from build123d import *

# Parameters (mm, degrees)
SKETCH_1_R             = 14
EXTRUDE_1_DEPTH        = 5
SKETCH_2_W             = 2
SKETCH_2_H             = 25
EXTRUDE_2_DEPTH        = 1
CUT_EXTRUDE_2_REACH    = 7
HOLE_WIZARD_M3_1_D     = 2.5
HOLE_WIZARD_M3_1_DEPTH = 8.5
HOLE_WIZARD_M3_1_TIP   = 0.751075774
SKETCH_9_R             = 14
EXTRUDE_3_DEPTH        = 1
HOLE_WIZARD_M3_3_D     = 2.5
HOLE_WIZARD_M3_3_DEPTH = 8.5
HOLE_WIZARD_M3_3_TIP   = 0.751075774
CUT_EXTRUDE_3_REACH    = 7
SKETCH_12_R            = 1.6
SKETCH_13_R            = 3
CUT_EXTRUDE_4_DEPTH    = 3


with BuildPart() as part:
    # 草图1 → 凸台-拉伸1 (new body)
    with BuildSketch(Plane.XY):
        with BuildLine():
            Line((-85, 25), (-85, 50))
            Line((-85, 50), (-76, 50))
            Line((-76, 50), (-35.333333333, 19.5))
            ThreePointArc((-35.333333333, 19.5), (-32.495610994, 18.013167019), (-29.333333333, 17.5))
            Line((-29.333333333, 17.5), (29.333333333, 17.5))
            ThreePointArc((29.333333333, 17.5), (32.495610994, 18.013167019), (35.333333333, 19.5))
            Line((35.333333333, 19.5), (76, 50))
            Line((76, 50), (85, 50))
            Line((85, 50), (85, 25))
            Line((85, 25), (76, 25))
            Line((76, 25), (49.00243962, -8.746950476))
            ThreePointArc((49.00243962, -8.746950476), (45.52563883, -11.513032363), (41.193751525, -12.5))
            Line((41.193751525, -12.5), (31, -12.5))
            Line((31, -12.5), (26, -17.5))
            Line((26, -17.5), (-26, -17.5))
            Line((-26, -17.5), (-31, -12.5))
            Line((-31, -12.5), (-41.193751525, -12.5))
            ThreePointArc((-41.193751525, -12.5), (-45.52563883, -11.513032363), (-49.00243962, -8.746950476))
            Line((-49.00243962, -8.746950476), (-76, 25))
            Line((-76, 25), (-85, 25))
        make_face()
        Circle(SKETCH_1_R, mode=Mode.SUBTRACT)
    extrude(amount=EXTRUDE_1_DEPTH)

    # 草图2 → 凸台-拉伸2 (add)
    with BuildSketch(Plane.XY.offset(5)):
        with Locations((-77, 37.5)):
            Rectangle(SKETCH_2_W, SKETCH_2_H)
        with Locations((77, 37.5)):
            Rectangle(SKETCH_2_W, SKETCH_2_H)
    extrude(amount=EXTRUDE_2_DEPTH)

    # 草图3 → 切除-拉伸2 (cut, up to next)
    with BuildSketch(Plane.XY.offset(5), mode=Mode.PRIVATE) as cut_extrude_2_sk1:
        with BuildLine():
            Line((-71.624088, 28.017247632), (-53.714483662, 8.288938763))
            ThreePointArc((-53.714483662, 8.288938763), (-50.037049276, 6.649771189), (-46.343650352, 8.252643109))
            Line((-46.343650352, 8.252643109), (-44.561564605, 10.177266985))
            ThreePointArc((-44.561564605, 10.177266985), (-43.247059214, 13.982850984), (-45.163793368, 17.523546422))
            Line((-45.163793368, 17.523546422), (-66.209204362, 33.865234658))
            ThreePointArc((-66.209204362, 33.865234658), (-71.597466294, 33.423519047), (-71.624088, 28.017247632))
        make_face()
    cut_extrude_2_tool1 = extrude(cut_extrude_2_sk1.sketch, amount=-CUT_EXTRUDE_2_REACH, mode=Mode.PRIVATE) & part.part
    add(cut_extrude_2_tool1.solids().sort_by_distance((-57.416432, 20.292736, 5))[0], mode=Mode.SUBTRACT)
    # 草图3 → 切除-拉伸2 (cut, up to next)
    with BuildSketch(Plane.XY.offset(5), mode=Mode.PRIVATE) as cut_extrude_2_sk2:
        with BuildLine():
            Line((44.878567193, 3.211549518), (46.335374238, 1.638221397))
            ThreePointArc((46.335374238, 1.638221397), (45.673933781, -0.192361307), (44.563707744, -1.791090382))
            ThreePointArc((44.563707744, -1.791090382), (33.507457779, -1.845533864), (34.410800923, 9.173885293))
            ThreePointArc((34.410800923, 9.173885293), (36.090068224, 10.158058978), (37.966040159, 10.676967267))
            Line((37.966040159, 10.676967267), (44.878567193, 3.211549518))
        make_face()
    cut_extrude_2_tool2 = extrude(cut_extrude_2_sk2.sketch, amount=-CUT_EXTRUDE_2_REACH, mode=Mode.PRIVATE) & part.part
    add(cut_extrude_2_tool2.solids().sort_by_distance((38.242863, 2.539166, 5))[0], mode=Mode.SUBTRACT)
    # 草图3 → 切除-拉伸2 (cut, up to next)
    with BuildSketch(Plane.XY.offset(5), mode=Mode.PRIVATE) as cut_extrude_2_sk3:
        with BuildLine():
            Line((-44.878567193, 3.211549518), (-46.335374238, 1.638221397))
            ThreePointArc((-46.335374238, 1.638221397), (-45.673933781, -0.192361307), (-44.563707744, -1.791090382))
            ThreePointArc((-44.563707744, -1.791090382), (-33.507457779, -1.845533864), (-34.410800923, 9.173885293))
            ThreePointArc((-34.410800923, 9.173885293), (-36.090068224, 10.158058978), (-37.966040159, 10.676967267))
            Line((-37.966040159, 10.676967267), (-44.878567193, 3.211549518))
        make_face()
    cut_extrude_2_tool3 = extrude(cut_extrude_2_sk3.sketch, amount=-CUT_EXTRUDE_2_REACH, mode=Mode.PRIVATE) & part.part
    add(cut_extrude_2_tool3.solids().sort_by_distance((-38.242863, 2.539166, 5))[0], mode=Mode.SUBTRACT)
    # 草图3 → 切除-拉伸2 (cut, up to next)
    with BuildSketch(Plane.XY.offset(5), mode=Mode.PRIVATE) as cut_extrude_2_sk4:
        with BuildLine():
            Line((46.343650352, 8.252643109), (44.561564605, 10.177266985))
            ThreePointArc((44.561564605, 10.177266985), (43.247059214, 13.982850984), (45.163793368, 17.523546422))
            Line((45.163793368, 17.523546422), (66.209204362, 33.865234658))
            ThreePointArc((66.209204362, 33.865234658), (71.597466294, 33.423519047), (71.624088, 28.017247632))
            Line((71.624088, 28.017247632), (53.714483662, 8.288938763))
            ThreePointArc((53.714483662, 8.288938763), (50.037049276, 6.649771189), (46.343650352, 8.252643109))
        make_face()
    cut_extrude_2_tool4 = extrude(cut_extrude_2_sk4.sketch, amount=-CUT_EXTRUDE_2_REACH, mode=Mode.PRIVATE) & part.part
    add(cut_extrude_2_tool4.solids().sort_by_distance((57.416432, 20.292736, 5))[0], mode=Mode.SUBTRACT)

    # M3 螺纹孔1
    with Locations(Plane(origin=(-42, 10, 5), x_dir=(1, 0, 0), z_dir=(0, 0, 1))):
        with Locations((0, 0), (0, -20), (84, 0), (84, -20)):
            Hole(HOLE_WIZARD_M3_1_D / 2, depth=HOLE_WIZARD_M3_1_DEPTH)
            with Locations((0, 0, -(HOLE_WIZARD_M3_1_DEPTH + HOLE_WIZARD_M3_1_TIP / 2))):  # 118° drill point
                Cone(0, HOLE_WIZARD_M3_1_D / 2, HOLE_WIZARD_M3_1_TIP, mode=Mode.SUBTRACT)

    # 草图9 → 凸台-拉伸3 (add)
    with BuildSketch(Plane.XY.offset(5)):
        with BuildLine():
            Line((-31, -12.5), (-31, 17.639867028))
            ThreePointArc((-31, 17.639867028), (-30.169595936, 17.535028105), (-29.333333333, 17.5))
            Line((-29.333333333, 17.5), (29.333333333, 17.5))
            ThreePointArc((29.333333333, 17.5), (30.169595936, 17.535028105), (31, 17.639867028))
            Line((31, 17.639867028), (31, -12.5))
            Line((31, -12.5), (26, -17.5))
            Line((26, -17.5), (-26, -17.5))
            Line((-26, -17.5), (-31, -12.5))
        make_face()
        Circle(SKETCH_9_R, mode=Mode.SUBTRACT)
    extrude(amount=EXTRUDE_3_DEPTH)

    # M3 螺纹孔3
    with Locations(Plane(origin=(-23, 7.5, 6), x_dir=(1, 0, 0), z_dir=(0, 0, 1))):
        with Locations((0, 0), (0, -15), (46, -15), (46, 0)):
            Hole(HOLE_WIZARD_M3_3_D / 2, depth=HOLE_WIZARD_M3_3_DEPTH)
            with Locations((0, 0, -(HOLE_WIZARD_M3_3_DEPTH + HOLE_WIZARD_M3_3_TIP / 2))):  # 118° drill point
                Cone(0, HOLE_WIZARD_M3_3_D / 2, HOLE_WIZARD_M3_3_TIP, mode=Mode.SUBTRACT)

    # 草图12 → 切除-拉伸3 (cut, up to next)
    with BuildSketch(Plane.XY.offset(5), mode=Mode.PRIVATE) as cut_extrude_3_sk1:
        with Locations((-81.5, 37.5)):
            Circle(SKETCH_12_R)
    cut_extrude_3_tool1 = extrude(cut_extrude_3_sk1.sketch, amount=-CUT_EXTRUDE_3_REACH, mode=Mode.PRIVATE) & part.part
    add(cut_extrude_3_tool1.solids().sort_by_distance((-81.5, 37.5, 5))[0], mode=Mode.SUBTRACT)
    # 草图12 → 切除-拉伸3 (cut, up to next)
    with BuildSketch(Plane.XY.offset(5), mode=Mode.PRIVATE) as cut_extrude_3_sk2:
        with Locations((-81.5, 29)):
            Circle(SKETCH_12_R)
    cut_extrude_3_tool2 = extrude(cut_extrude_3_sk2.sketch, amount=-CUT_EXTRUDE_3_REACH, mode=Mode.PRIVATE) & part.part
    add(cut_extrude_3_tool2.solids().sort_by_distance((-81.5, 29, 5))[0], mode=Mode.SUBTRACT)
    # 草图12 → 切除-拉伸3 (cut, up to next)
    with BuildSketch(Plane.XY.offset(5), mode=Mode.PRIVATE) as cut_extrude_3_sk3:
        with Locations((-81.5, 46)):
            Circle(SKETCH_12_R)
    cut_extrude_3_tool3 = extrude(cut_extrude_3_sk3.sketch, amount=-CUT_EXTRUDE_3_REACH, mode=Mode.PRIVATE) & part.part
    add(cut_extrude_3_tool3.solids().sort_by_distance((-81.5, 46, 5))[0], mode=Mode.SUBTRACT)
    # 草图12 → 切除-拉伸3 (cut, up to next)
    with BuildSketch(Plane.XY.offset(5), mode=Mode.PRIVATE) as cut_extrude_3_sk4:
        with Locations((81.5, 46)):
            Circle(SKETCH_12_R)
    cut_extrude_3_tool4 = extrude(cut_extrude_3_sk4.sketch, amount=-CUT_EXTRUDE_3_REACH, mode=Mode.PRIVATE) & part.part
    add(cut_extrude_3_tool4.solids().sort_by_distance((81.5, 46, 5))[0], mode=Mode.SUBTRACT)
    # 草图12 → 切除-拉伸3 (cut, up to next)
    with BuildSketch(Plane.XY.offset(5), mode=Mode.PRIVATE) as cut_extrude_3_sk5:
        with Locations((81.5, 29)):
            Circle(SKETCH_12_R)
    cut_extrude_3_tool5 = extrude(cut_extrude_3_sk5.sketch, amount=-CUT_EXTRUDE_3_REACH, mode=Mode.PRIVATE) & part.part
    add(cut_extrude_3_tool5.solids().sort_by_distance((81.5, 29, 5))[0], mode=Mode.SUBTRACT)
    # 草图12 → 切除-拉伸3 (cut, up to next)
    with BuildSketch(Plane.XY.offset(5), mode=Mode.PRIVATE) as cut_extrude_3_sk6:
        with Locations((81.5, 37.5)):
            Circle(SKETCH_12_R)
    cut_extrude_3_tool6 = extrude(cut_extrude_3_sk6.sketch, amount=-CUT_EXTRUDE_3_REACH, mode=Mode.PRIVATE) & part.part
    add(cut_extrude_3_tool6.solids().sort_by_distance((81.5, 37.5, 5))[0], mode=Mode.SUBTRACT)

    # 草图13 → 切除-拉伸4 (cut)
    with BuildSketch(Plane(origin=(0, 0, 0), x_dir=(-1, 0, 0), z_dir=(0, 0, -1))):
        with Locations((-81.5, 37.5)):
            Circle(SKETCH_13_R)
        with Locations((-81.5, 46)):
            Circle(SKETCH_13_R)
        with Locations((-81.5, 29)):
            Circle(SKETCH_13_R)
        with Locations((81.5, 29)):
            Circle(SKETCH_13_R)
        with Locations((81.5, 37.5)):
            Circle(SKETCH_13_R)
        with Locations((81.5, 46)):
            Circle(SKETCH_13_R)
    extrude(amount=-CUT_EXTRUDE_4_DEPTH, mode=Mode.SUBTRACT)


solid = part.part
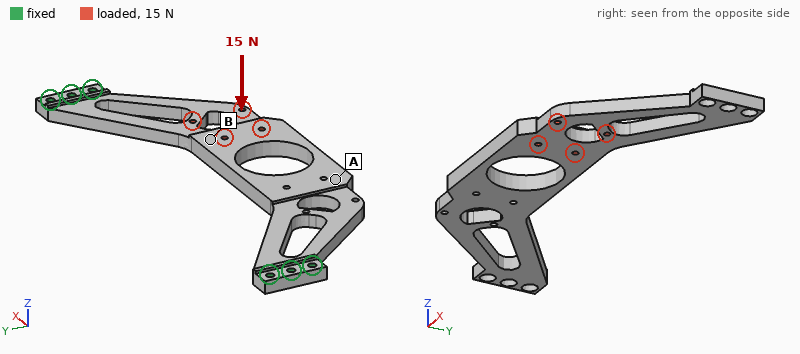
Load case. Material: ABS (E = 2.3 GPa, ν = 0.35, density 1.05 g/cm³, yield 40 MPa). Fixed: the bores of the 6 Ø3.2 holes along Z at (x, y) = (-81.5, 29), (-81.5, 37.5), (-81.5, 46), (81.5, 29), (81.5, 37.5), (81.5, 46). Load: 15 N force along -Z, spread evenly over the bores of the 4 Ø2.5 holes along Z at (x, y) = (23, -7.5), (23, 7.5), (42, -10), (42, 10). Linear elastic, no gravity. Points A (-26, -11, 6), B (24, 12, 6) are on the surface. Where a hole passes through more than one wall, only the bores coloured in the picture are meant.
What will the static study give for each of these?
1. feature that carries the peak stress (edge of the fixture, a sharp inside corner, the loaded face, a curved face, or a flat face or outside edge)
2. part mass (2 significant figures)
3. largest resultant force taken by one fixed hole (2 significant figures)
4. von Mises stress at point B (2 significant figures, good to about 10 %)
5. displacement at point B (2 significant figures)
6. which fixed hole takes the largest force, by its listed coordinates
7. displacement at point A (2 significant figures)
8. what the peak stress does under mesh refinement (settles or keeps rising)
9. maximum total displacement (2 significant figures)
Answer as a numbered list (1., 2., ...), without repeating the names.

1. edge of the fixture
2. 22 g
3. 27 N
4. 1.5 MPa
5. 0.94 mm
6. (81.5, 29)
7. 1.2 mm
8. keeps rising
9. 1.7 mm
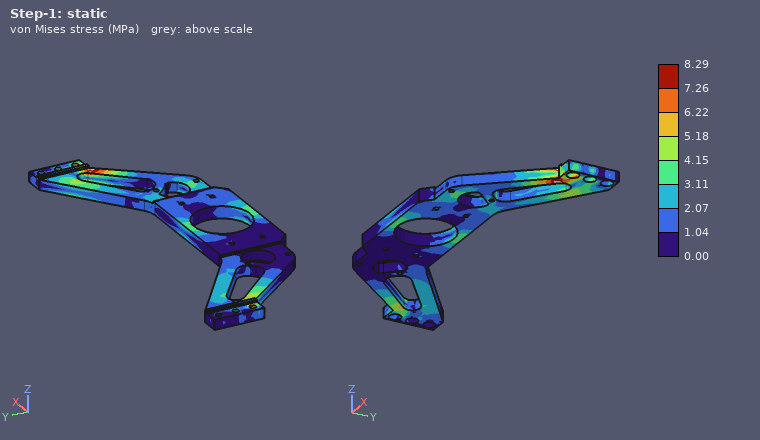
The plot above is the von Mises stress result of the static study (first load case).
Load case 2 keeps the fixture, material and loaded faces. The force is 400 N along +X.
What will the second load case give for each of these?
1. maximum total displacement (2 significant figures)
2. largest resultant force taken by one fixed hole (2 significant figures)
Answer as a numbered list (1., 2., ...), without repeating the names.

1. 0.53 mm
2. 97 N
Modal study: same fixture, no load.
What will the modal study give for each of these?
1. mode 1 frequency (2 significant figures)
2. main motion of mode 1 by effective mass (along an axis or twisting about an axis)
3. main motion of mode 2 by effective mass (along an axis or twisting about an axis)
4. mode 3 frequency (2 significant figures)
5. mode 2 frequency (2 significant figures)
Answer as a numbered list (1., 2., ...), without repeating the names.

1. 150 Hz
2. along Z
3. twisting about Y
4. 570 Hz
5. 470 Hz
